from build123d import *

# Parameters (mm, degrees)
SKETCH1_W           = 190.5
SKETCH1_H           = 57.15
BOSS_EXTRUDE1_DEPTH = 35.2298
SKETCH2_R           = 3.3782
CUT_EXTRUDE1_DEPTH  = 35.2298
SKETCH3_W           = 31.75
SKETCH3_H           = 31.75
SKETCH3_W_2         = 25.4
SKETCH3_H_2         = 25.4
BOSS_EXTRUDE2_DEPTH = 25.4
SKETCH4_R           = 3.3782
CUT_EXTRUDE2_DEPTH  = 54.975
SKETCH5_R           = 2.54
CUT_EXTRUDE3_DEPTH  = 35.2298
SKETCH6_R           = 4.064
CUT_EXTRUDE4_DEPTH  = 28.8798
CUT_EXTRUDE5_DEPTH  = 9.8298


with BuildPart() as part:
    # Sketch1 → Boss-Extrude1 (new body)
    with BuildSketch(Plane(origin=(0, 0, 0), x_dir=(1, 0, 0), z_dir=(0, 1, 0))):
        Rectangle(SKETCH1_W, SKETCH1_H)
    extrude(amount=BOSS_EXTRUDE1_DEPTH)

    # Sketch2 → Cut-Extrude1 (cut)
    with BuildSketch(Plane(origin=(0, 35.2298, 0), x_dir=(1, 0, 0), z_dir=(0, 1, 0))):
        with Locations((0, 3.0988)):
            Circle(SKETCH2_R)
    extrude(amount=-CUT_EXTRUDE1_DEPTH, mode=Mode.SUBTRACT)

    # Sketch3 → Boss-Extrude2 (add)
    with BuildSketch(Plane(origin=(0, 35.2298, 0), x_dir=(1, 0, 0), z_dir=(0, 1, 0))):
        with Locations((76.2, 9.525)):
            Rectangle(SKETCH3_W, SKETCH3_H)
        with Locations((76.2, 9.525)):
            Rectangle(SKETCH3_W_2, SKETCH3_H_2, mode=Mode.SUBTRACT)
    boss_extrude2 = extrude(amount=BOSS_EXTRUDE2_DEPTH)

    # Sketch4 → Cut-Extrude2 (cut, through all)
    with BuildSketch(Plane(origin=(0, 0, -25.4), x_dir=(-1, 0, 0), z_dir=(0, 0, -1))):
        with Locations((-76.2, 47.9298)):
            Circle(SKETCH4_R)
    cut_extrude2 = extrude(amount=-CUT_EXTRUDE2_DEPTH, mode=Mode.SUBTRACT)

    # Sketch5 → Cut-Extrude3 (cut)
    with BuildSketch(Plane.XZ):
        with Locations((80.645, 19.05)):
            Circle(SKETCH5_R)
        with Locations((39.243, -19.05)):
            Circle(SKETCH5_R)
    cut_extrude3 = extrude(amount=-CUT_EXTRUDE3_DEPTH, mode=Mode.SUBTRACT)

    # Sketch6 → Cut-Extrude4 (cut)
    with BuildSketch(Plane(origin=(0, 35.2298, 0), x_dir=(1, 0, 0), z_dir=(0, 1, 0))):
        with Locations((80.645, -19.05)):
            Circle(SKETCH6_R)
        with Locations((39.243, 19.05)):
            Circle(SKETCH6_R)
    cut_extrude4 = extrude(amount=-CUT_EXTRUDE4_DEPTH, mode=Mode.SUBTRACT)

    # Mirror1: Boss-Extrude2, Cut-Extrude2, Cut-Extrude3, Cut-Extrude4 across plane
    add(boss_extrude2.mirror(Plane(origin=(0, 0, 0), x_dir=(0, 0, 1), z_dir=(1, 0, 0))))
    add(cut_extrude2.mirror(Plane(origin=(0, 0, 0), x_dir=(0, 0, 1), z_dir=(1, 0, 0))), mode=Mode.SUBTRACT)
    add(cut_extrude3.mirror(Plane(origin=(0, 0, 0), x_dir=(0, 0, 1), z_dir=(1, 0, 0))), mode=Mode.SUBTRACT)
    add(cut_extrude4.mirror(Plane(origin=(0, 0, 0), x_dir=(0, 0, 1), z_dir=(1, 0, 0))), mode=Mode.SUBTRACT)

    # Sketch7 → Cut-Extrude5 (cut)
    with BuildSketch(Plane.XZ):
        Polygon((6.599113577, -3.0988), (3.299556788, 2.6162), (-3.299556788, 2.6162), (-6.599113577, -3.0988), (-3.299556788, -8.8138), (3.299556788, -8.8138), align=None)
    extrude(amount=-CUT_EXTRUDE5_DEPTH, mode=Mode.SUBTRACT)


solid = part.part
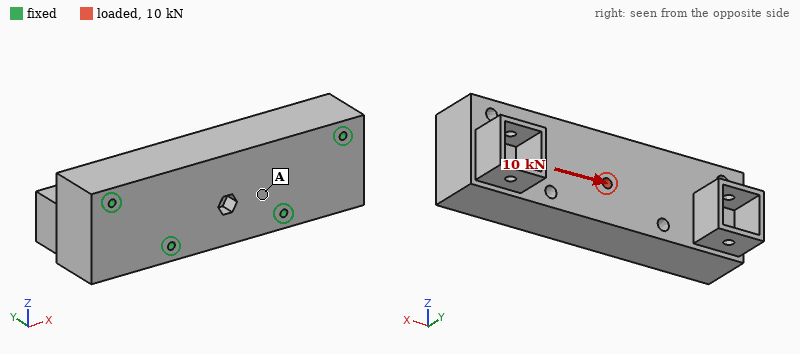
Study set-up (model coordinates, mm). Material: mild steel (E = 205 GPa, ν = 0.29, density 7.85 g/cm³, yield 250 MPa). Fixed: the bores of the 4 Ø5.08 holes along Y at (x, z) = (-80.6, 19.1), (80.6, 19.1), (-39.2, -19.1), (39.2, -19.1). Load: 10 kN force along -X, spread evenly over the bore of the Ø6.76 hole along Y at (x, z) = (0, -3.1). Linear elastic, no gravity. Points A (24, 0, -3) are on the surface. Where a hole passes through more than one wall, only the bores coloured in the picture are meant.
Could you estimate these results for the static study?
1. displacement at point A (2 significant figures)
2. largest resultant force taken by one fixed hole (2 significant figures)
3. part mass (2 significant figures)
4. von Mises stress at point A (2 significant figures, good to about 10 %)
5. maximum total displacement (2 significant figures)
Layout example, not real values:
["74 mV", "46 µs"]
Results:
["1.3 µm", "3.1 kN", "3.1 kg", "4.6 MPa", "3.0 µm"]
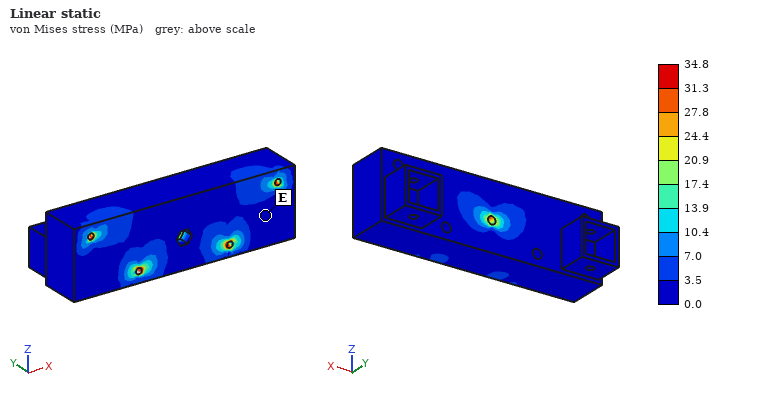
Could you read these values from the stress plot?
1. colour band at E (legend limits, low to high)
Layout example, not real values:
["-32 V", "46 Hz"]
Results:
["0.0 to 3.5 MPa"]
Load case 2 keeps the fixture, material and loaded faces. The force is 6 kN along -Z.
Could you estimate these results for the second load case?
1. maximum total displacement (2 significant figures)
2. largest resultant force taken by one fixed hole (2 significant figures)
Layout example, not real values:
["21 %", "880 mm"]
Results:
["7.0 µm", "2.8 kN"]
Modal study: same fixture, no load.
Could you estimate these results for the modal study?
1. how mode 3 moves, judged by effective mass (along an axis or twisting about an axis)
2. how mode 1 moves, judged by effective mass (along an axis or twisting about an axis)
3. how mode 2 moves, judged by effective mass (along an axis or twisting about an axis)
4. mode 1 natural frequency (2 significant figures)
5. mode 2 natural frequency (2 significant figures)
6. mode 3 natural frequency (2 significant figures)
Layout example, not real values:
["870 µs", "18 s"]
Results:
["along Y", "along Z", "along X", "3400 Hz", "5000 Hz", "6700 Hz"]
